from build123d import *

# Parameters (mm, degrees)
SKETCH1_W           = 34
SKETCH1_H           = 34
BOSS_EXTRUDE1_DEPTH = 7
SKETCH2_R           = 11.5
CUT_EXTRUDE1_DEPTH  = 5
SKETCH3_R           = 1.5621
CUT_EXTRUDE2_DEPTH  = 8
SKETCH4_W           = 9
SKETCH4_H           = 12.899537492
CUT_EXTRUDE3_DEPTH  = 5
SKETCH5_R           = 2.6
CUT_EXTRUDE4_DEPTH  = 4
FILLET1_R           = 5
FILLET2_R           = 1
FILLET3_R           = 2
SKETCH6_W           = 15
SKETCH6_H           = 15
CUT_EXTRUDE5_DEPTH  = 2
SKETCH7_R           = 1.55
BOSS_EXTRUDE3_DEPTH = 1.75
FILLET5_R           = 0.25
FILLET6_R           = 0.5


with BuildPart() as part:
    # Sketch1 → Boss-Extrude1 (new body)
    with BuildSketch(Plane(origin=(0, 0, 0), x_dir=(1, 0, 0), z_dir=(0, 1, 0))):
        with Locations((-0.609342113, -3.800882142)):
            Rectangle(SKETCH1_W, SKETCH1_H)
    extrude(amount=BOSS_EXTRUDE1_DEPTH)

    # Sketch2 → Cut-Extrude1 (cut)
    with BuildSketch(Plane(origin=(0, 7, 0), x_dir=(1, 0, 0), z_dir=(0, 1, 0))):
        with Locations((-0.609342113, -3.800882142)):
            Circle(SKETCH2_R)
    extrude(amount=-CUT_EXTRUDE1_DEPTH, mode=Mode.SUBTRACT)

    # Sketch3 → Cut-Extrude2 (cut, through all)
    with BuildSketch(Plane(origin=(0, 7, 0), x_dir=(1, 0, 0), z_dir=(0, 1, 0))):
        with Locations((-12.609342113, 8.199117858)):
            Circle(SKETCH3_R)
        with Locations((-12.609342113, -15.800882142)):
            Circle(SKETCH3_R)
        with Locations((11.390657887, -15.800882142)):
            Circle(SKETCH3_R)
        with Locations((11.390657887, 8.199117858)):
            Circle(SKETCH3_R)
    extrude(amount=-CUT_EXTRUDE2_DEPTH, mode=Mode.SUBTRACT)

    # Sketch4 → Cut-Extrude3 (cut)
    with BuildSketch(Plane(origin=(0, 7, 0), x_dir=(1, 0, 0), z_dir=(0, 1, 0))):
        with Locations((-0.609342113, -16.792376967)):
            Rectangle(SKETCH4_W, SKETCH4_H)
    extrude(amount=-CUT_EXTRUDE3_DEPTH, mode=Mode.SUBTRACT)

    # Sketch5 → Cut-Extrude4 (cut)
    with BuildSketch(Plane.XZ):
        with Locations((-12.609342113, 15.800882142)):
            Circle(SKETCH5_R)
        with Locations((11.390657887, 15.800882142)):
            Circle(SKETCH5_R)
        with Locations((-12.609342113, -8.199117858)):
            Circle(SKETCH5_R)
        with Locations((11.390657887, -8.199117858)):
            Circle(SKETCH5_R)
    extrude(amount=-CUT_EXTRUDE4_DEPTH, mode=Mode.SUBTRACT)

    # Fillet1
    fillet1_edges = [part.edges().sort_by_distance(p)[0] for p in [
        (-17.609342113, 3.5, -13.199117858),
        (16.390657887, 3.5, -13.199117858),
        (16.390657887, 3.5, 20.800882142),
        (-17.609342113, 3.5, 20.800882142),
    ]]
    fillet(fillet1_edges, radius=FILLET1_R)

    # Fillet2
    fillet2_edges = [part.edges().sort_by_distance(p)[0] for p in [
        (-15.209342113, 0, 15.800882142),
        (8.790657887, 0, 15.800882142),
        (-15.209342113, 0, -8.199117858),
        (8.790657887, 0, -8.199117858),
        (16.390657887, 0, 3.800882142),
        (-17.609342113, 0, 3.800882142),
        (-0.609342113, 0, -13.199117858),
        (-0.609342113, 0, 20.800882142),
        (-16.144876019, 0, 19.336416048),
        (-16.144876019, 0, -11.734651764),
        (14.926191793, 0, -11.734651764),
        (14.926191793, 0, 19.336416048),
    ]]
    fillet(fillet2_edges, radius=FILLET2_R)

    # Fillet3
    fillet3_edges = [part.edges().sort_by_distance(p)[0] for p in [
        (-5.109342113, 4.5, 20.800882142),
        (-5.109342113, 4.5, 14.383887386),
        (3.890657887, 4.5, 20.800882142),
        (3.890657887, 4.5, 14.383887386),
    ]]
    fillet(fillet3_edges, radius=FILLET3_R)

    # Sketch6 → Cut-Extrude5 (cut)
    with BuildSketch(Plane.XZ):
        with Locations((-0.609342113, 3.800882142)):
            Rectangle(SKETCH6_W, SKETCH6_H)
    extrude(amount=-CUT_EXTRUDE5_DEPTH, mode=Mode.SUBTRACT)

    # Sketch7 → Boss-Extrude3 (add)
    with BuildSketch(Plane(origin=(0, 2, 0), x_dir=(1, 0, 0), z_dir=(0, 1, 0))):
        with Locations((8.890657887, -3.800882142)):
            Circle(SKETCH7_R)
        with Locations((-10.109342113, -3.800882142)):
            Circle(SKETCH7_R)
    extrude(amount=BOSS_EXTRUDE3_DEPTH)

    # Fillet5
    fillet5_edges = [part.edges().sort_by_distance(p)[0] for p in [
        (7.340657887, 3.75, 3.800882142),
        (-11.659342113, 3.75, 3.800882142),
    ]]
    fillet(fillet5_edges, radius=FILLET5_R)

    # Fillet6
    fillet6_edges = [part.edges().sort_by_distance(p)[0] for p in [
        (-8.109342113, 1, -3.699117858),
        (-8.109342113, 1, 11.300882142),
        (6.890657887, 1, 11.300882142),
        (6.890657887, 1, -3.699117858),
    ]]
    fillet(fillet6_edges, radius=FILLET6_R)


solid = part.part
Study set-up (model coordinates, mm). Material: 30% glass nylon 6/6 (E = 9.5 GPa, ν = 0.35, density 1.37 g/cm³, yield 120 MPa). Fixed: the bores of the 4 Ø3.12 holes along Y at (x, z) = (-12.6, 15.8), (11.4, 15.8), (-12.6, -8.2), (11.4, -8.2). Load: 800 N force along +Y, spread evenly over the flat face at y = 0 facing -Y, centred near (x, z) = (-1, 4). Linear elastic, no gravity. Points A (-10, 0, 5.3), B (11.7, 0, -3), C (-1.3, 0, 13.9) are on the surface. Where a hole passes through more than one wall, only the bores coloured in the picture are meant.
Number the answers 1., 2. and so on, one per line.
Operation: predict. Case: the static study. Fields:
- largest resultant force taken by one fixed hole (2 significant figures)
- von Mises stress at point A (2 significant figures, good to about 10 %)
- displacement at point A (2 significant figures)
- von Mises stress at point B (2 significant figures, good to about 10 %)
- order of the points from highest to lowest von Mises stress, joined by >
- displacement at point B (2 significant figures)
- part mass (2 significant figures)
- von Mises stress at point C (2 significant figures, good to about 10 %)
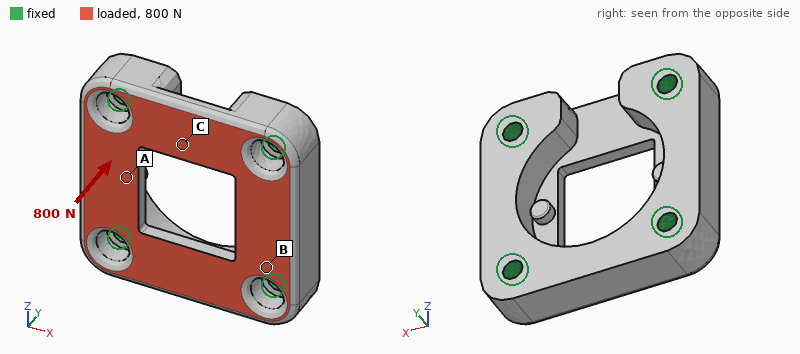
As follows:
1. 230 N
2. 9.0 MPa
3. 22 µm
4. 3.2 MPa
5. C > A > B
6. 9.6 µm
7. 6.4 g
8. 16 MPa
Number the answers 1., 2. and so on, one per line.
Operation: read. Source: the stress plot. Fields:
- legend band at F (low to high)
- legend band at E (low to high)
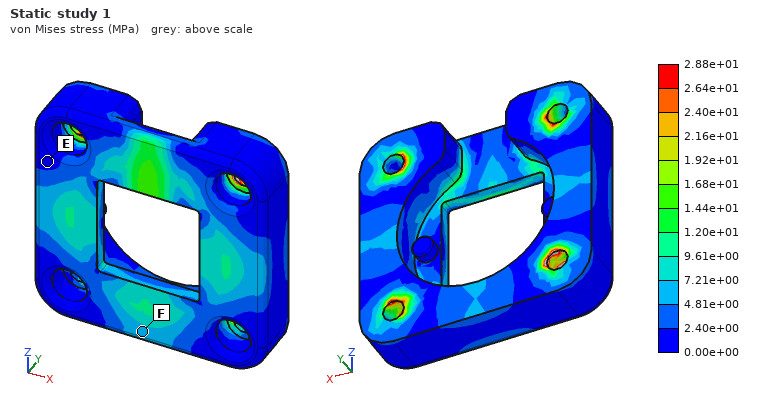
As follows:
1. 4.81e+00 to 7.21e+00 MPa
2. 0.00e+00 to 2.40e+00 MPa
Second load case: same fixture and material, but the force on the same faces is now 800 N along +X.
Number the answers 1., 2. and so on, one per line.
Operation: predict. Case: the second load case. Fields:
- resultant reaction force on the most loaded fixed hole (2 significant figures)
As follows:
1. 220 N
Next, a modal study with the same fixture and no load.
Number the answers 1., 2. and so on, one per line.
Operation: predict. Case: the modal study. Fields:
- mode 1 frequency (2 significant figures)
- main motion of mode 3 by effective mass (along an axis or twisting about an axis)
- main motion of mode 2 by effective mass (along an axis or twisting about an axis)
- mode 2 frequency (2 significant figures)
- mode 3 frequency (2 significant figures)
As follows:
1. 16 kHz
2. along Y
3. along X
4. 18 kHz
5. 19 kHz
